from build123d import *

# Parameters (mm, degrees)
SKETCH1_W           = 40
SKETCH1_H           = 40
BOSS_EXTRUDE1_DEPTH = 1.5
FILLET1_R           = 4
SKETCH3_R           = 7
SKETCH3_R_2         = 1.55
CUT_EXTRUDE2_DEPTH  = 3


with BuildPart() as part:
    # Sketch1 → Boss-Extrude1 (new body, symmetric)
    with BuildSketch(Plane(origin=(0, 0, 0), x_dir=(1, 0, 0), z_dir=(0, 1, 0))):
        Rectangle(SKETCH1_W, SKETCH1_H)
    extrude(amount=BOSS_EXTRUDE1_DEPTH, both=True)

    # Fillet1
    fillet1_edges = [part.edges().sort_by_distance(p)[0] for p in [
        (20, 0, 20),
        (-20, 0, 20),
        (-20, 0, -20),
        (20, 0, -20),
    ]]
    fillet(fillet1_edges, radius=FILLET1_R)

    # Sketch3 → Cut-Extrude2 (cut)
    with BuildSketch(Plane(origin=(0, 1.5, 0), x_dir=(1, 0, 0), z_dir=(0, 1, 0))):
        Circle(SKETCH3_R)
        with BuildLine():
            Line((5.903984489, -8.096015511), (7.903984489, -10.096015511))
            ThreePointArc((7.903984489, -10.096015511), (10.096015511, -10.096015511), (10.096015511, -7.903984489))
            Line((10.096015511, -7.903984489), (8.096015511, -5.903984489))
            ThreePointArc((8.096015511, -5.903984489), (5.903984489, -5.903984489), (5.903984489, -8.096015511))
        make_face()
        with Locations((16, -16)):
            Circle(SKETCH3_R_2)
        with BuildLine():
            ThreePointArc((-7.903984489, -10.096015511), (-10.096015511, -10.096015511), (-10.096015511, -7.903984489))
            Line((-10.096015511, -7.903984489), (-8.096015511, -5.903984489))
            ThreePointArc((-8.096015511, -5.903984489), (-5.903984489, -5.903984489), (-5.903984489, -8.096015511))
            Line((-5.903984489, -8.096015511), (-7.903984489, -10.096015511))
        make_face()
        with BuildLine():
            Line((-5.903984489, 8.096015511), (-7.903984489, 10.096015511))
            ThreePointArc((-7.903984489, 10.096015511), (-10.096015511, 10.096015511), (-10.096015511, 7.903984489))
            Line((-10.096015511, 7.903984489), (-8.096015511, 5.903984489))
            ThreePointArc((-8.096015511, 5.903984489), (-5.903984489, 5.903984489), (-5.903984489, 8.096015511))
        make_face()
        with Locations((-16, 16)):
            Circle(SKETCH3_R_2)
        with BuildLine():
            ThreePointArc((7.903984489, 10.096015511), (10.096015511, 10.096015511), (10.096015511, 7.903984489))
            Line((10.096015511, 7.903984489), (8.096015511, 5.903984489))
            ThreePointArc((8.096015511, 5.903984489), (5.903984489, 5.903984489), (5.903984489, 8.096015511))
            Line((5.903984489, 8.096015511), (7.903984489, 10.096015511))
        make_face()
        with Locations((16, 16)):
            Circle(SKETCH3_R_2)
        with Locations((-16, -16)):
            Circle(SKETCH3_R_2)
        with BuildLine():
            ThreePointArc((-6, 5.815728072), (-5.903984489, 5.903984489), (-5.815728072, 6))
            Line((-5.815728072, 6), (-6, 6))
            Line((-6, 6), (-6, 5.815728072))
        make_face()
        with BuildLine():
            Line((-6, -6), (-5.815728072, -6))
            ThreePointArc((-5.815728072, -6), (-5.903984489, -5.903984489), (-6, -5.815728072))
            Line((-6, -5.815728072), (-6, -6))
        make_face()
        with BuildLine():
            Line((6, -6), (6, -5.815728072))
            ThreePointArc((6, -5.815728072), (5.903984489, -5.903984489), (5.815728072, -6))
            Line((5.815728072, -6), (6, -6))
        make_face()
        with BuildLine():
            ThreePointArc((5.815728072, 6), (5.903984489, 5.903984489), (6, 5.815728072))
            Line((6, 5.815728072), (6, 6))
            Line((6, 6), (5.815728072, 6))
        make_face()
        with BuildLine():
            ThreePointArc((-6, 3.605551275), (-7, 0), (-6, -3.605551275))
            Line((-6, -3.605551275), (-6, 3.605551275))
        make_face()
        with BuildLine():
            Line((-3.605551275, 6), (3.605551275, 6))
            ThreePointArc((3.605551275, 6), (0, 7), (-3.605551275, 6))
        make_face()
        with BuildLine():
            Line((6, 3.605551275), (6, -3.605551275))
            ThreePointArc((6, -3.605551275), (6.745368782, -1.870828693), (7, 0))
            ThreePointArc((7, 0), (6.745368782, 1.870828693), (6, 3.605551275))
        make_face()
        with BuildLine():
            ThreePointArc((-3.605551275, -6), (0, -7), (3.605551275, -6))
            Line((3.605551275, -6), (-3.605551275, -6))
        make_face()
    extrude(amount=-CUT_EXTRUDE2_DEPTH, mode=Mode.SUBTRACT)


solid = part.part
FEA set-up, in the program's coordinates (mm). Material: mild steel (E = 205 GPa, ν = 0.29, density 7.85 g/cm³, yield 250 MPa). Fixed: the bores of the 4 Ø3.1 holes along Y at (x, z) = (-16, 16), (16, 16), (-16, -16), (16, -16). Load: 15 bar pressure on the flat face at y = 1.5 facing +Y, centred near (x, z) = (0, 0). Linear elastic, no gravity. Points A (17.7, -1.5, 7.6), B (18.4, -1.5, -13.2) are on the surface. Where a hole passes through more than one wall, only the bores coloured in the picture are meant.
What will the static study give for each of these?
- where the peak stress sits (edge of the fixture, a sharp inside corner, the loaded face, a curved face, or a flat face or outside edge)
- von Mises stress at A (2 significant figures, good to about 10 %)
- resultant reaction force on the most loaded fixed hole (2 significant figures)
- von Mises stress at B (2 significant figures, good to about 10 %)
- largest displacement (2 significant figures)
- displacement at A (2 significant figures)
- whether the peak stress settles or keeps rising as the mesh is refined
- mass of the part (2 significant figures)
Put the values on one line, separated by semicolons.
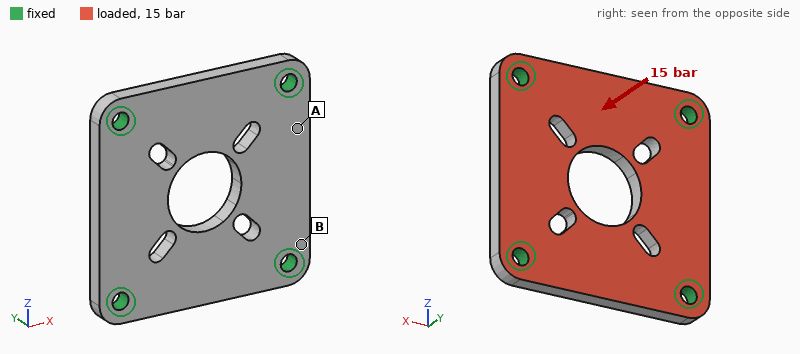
edge of the fixture; 18 MPa; 500 N; 53 MPa; 19 µm; 5.4 µm; keeps rising; 31 g
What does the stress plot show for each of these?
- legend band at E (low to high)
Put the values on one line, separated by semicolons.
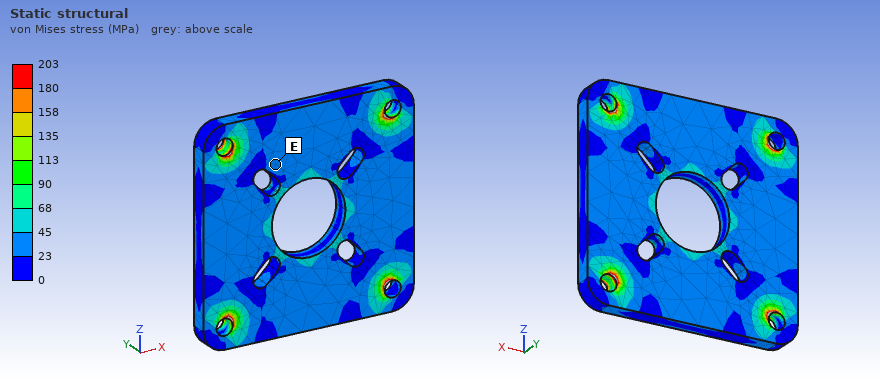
23 to 45 MPa
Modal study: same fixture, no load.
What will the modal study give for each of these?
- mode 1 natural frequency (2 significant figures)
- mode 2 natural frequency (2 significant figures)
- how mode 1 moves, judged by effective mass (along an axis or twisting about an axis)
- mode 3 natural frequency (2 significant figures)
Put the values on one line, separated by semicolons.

11 kHz; 16 kHz; along Y; 16 kHz
